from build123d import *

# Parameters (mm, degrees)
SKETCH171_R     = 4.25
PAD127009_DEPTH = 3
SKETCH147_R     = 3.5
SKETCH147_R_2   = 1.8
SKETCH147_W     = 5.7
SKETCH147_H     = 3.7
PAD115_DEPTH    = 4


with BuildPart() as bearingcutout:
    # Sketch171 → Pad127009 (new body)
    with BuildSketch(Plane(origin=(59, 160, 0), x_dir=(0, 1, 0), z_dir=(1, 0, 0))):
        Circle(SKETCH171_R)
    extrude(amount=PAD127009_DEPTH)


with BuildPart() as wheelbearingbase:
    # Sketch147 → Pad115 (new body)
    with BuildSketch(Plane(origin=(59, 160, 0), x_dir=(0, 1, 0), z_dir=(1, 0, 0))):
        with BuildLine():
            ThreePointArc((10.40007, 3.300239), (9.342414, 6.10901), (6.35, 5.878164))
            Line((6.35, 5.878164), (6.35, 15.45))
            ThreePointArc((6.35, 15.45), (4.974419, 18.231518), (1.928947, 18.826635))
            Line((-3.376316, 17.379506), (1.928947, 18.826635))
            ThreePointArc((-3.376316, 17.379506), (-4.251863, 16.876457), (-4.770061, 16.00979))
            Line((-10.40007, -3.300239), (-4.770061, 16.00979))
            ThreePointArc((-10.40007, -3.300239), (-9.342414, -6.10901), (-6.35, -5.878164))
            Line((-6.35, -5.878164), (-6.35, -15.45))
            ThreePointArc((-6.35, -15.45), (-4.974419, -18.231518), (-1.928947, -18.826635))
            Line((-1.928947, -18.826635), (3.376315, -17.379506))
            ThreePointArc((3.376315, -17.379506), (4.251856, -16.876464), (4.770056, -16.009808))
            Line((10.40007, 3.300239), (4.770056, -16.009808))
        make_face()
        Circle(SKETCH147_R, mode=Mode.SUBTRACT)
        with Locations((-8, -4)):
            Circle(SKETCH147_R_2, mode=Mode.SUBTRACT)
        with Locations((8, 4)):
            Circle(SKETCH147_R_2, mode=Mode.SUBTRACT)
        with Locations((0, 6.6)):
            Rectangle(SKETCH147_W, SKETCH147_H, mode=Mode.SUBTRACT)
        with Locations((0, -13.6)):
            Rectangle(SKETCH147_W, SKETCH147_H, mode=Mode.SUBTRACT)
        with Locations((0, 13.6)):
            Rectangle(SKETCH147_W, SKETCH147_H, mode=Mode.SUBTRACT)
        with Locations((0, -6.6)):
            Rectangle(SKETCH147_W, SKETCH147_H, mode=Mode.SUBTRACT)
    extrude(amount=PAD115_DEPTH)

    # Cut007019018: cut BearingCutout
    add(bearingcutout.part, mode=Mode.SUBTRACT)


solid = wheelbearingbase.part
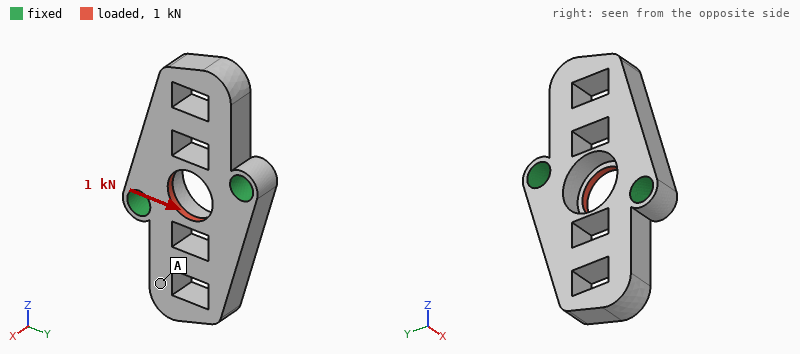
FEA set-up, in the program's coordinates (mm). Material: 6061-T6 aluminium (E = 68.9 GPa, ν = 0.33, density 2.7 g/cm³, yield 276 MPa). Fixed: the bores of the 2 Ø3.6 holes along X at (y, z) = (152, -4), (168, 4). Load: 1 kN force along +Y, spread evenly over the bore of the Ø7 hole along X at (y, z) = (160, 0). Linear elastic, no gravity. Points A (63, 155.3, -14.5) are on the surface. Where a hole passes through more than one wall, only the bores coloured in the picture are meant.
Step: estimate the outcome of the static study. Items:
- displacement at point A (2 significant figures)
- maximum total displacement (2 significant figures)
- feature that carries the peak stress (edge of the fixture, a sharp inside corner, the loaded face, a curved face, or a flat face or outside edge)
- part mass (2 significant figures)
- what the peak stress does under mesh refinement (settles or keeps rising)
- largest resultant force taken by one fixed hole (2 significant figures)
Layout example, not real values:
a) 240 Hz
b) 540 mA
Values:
a) 2.2 µm
b) 5.6 µm
c) a sharp inside corner
d) 4.0 g
e) keeps rising
f) 500 N
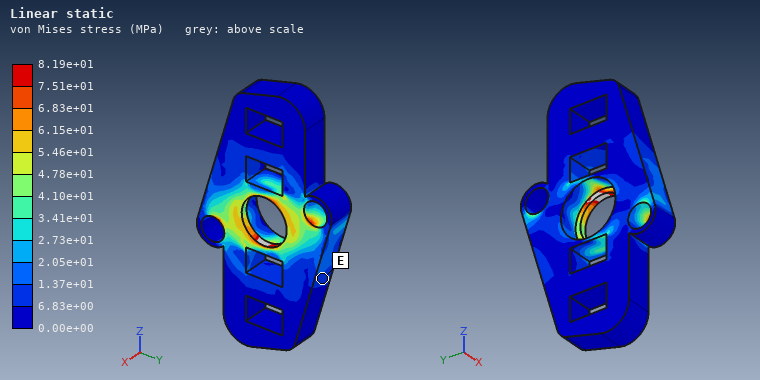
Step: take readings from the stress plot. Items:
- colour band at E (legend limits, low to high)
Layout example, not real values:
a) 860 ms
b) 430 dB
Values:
a) 6.83e+00 to 1.37e+01 MPa
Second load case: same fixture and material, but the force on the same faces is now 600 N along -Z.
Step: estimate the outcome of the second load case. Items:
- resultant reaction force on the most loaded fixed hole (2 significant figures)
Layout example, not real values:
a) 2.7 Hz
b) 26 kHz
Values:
a) 300 N
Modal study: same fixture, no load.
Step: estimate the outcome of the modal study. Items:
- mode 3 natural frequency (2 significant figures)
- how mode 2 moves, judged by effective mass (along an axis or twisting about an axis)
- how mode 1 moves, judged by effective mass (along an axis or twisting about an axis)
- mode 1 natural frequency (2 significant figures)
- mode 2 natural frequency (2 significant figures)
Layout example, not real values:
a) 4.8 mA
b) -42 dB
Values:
a) 24 kHz
b) along X
c) twisting about Y
d) 10 kHz
e) 11 kHz
